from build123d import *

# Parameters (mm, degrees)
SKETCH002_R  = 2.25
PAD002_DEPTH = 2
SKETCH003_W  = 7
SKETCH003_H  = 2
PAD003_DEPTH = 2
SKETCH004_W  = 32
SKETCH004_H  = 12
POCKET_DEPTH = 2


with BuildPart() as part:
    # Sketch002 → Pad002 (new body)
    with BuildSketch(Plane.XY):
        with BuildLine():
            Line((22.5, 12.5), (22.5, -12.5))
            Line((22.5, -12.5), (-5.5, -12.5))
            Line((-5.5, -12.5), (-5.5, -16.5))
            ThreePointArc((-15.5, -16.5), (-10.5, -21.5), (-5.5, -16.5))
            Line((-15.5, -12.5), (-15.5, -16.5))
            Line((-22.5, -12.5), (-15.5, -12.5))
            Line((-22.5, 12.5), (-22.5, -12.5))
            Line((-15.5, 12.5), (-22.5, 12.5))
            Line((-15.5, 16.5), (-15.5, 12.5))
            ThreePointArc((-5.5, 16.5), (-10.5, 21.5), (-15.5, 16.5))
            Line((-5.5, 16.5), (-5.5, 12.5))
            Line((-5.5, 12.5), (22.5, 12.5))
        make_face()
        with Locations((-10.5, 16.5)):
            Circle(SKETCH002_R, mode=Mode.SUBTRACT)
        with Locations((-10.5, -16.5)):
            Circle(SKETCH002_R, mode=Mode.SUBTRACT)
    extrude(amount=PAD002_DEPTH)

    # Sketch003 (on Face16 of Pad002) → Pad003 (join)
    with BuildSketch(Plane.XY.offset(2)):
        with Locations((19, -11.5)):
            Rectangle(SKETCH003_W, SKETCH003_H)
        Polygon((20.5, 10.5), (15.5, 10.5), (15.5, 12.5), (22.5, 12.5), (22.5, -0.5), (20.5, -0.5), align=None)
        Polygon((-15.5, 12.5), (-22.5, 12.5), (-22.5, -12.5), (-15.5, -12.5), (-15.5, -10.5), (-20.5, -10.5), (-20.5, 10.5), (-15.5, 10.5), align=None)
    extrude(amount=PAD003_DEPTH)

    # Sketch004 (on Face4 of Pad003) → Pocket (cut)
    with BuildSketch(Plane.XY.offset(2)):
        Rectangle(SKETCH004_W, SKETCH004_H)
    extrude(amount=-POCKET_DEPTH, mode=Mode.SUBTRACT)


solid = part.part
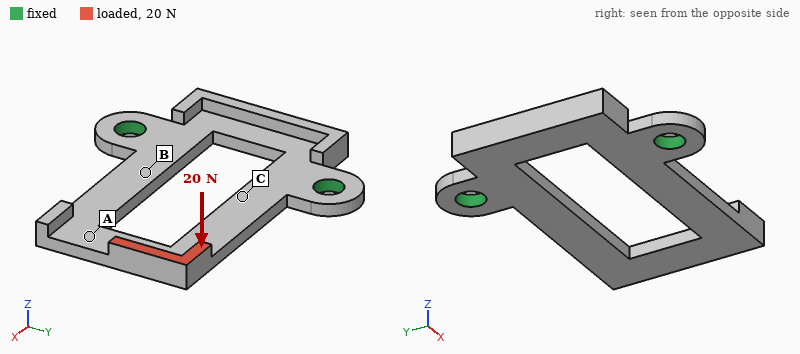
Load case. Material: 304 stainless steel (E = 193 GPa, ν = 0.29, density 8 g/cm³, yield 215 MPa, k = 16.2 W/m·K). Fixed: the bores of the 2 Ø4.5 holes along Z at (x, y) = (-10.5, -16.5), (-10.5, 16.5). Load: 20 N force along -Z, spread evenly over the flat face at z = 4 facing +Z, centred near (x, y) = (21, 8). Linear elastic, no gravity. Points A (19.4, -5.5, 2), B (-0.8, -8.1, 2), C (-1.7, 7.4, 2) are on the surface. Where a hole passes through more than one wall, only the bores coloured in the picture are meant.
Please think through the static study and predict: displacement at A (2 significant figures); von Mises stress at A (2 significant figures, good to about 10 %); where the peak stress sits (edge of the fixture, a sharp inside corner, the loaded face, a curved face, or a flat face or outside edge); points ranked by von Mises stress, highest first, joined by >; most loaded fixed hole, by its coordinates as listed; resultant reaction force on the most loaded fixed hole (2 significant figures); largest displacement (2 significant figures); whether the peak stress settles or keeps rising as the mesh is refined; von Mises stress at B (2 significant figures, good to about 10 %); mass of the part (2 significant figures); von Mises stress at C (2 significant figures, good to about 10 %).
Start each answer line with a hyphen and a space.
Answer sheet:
- 0.10 mm
- 12 MPa
- a sharp inside corner
- C > B > A
- (-10.5, 16.5)
- 15 N
- 0.14 mm
- keeps rising
- 43 MPa
- 16 g
- 58 MPa
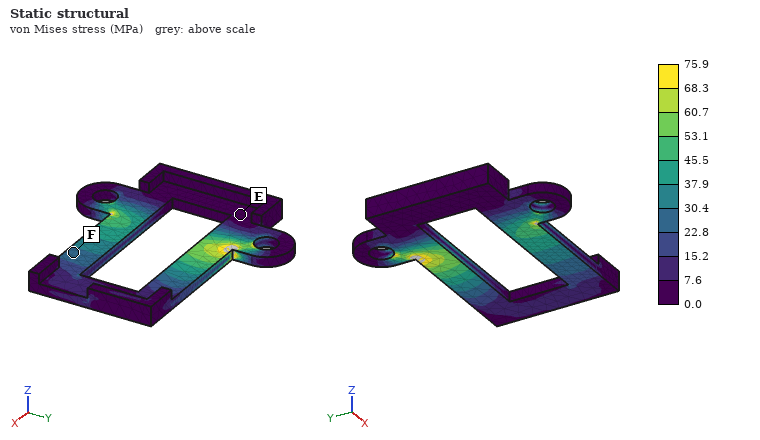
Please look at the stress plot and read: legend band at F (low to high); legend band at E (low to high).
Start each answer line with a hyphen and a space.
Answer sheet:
- 22.8 to 30.4 MPa
- 0.0 to 7.6 MPa
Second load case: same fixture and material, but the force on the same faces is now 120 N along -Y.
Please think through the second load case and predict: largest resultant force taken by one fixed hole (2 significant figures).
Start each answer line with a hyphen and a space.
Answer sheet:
- 120 N
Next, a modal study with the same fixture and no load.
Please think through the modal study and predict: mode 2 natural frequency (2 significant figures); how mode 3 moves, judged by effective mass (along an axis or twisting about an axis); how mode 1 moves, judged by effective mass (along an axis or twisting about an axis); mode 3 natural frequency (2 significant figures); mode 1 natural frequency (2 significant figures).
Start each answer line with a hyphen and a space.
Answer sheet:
- 3200 Hz
- along Z
- along Z
- 6100 Hz
- 1100 Hz
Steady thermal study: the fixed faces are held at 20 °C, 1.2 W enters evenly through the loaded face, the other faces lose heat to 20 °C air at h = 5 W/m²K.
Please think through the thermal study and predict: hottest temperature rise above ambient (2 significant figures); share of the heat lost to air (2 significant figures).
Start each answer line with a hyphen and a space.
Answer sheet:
- 85 K
- 27 %
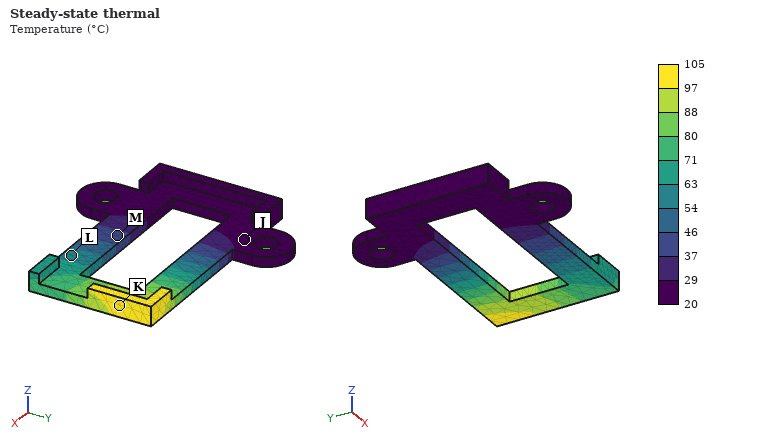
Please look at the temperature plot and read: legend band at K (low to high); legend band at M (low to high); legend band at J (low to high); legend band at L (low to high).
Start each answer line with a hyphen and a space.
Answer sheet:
- 97 to 105 °C
- 37 to 46 °C
- 20 to 29 °C
- 54 to 63 °C
